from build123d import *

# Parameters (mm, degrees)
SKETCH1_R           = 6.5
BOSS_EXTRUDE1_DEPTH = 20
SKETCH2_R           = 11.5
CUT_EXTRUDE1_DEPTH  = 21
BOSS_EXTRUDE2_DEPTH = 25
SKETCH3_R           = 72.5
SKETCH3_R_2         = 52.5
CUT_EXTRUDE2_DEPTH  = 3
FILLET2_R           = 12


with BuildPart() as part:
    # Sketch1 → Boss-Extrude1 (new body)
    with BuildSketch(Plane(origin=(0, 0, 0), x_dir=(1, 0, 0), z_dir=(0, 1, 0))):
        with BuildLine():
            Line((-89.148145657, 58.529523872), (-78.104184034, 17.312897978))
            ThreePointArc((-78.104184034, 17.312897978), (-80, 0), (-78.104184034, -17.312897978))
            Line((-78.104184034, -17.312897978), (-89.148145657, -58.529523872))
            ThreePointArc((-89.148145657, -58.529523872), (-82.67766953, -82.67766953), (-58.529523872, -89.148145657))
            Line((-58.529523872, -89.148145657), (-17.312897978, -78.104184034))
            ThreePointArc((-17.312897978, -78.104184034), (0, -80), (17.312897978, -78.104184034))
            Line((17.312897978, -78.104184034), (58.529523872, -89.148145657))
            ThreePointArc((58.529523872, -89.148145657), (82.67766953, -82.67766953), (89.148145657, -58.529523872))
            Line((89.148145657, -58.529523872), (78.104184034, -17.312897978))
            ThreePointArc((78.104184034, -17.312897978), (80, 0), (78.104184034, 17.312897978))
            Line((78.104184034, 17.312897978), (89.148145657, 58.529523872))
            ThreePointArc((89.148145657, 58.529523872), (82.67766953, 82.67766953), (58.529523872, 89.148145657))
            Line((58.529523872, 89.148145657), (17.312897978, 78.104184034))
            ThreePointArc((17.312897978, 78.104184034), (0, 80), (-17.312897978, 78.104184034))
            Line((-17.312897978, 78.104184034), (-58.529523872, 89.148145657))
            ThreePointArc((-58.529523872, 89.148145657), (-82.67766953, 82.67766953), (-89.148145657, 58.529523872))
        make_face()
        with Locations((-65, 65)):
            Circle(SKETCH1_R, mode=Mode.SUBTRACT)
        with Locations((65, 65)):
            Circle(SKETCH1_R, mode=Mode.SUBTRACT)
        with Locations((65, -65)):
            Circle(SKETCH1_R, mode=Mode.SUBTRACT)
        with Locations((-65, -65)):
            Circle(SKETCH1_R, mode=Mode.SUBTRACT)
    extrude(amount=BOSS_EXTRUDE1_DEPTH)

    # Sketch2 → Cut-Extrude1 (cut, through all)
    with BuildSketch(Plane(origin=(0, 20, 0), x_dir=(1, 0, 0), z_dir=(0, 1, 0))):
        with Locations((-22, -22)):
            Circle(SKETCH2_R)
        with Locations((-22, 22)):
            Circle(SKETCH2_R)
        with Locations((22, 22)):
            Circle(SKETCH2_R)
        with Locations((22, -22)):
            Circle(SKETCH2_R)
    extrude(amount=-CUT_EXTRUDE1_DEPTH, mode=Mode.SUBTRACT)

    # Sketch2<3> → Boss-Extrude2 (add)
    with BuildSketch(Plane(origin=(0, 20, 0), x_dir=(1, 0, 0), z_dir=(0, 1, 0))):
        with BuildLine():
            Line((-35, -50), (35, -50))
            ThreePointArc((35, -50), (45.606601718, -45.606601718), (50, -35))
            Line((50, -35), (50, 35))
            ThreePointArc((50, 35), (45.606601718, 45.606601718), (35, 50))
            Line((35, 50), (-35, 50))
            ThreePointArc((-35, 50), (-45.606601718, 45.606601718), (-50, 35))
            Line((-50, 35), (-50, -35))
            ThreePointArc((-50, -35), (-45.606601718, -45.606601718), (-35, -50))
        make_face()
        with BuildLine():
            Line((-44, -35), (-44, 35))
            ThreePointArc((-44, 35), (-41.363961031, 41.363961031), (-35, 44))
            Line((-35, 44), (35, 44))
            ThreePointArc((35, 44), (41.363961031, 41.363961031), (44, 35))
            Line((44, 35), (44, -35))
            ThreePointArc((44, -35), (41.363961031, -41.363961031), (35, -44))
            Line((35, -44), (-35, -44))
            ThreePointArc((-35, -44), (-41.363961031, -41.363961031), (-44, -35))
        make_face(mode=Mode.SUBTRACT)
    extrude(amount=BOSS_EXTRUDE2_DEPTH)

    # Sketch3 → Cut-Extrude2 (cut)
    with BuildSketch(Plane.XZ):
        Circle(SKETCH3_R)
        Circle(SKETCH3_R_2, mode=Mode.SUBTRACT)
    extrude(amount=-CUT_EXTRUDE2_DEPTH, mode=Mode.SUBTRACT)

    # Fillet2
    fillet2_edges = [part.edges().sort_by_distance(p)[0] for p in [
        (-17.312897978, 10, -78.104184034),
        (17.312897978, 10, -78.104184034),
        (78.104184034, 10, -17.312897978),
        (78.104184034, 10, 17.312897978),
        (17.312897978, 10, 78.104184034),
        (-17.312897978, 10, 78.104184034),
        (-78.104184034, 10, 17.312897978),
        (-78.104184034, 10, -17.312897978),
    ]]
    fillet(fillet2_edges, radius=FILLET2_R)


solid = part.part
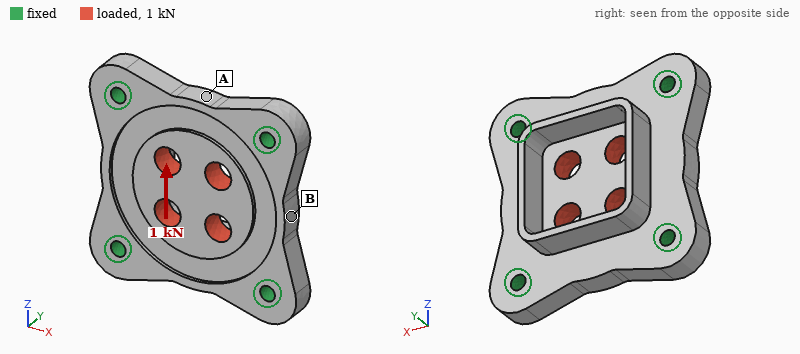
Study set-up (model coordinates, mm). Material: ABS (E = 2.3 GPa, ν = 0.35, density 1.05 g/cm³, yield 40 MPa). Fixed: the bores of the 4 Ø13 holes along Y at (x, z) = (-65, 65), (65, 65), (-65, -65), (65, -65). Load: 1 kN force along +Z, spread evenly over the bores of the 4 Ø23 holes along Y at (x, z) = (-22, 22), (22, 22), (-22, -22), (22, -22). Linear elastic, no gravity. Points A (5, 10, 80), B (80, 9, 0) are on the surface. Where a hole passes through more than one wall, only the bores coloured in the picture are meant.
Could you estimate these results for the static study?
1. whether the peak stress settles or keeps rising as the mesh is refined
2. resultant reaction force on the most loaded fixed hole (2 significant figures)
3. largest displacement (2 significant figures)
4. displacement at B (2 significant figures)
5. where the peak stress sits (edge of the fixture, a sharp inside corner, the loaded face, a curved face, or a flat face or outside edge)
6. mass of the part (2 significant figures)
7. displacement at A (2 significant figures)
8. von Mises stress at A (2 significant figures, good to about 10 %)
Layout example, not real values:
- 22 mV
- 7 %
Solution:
- keeps rising
- 280 N
- 16 µm
- 3.3 µm
- edge of the fixture
- 580 g
- 12 µm
- 0.24 MPa
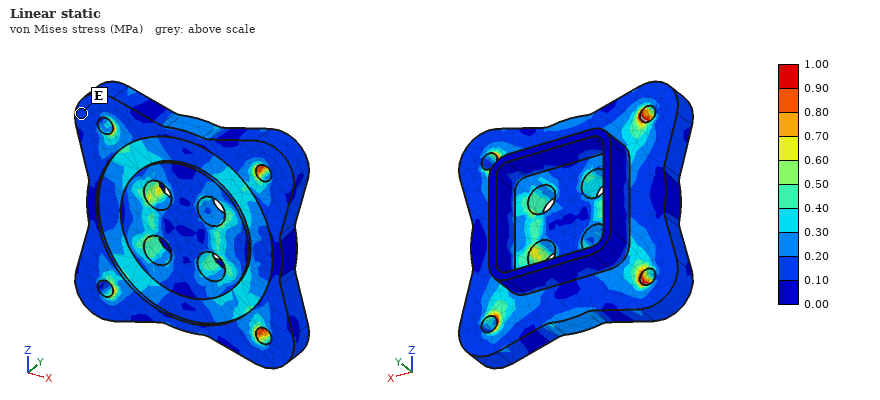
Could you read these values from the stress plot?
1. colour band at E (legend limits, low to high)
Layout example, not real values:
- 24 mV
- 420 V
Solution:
- 0.10 to 0.20 MPa
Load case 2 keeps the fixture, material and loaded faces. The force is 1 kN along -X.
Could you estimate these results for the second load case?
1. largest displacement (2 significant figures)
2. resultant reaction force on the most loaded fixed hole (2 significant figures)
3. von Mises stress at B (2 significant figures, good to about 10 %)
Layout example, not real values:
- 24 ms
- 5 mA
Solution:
- 16 µm
- 280 N
- 0.23 MPa
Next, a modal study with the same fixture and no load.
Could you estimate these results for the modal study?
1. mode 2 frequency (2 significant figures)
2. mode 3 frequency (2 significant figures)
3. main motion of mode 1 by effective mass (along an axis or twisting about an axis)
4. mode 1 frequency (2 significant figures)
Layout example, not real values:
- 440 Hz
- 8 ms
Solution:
- 1800 Hz
- 1800 Hz
- along Y
- 1200 Hz
